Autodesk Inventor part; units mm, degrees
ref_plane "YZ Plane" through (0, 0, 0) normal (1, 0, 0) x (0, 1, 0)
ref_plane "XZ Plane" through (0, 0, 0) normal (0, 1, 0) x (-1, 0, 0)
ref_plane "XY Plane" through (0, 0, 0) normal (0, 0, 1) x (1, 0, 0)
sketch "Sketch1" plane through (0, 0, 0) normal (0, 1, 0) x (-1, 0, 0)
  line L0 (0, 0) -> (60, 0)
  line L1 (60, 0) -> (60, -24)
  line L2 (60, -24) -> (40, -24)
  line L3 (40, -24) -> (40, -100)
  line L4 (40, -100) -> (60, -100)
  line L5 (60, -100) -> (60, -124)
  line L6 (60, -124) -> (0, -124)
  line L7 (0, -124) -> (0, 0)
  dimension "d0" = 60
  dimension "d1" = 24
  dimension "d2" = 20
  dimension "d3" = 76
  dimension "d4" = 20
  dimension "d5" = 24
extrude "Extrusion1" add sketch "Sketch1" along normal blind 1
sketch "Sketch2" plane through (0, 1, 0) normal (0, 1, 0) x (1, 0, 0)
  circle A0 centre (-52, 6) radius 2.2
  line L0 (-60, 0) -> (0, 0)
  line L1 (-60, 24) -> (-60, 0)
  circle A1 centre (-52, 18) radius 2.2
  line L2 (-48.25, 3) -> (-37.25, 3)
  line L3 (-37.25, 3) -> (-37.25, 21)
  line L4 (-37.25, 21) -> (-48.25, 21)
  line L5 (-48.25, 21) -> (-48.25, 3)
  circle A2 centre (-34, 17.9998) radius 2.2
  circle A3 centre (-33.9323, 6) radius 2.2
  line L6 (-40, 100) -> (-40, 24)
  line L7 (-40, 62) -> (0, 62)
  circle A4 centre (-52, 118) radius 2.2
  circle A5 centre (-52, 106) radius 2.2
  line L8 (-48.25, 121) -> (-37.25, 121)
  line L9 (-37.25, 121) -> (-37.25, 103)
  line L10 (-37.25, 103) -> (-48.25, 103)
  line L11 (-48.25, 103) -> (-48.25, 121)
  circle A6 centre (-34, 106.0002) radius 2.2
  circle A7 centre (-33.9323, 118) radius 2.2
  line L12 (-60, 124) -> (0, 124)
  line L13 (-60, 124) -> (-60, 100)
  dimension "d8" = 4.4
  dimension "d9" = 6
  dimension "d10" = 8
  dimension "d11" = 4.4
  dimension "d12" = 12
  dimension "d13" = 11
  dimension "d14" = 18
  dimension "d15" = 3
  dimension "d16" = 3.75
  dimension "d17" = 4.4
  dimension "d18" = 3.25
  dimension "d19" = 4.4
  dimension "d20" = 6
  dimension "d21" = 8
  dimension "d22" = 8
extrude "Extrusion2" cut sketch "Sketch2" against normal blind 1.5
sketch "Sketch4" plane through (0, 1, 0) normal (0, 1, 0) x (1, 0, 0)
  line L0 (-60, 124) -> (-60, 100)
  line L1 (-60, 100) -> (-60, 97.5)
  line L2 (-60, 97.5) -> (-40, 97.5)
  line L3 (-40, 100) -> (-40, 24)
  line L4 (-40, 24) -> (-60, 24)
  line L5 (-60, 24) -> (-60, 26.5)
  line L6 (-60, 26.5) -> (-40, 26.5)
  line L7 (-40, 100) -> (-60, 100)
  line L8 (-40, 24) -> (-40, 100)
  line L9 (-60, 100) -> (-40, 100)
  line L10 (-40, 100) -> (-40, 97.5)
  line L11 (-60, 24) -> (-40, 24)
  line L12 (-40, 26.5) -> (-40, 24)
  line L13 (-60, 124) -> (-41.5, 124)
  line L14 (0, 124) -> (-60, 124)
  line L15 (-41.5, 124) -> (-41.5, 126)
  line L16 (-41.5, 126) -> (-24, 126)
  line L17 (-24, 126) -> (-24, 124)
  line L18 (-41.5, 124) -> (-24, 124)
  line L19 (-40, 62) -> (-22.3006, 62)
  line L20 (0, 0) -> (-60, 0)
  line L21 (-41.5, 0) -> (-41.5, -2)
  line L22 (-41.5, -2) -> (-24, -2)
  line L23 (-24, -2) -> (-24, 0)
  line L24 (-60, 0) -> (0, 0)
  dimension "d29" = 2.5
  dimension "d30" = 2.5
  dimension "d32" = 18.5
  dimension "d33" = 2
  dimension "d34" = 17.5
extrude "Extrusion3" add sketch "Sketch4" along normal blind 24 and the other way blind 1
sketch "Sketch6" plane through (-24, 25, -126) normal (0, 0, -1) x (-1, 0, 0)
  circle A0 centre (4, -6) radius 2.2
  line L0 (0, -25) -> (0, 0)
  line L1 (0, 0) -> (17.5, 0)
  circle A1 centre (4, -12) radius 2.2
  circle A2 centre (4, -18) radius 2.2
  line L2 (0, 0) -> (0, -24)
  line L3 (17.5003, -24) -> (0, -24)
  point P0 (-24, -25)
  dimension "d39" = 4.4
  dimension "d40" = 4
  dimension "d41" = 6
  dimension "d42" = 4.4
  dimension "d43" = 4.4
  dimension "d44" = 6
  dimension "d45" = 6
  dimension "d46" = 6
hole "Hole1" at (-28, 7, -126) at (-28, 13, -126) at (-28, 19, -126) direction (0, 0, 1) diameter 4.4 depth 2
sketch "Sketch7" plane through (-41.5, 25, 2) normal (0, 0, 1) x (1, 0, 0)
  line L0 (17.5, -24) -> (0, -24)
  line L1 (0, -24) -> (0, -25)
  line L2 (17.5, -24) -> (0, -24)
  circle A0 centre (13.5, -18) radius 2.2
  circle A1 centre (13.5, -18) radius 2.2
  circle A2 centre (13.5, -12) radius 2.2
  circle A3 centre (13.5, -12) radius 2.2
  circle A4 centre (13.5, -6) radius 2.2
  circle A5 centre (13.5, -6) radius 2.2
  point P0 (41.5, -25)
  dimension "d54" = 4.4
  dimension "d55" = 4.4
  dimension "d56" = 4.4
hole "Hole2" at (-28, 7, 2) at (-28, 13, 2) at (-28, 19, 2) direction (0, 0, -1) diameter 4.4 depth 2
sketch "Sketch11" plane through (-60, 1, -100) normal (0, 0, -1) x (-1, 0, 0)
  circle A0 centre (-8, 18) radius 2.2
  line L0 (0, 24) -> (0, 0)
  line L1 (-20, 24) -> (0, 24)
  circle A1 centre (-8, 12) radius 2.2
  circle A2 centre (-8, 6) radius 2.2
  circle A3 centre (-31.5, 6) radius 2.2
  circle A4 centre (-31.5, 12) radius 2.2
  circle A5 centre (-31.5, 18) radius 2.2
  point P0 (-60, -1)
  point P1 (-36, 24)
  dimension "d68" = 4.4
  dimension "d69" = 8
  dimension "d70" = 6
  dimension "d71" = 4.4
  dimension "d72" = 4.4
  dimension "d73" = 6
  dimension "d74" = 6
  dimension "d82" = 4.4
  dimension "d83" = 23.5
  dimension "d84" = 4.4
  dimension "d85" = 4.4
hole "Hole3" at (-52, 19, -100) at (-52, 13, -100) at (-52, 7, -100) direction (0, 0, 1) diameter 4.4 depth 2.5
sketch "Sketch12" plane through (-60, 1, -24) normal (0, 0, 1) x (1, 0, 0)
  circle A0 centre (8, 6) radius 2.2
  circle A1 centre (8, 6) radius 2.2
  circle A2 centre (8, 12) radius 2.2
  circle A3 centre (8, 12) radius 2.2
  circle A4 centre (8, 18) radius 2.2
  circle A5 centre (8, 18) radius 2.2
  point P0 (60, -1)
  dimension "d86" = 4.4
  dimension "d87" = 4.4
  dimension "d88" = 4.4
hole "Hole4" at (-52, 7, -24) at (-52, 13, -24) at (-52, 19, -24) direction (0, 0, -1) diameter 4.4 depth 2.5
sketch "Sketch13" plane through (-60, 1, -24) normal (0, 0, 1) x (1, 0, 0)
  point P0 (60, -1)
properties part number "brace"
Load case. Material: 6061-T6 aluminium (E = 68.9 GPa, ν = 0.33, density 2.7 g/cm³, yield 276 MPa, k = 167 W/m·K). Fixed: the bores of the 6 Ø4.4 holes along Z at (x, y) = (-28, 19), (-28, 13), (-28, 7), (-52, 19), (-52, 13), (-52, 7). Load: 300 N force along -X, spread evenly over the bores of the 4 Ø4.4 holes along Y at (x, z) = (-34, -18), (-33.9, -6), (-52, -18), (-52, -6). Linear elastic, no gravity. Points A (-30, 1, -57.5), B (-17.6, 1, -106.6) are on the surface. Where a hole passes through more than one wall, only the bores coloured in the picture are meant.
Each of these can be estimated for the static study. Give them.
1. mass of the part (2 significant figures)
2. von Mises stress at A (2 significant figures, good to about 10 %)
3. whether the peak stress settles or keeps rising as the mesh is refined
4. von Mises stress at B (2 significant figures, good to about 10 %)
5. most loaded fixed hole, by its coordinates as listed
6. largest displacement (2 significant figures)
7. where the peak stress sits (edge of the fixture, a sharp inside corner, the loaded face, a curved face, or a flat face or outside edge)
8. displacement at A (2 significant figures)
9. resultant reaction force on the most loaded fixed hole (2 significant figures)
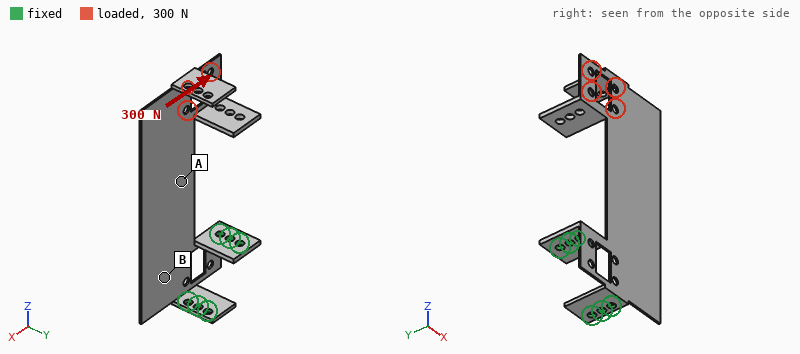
25 g
29 MPa
keeps rising
74 MPa
(-52, 7)
1.1 mm
a sharp inside corner
0.43 mm
1.5 kN
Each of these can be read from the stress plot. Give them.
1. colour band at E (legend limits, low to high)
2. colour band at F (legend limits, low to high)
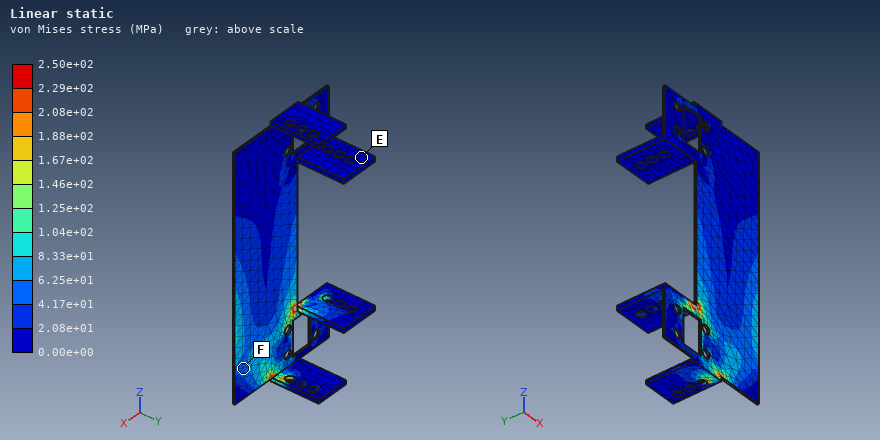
0.00e+00 to 2.08e+01 MPa
4.17e+01 to 6.25e+01 MPa
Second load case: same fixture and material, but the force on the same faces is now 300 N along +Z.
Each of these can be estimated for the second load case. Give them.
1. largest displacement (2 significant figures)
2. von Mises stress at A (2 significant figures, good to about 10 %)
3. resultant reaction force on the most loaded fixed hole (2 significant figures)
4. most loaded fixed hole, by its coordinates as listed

0.24 mm
21 MPa
200 N
(-28, 7)
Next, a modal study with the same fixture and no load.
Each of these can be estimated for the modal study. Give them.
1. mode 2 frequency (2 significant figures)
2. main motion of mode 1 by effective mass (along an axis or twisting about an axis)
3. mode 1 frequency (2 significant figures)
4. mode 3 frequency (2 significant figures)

140 Hz
along Y
44 Hz
260 Hz
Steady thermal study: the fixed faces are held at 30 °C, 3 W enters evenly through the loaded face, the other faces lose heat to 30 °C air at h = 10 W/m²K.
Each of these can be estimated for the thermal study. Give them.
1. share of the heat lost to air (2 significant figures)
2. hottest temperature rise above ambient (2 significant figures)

66 %
34 K
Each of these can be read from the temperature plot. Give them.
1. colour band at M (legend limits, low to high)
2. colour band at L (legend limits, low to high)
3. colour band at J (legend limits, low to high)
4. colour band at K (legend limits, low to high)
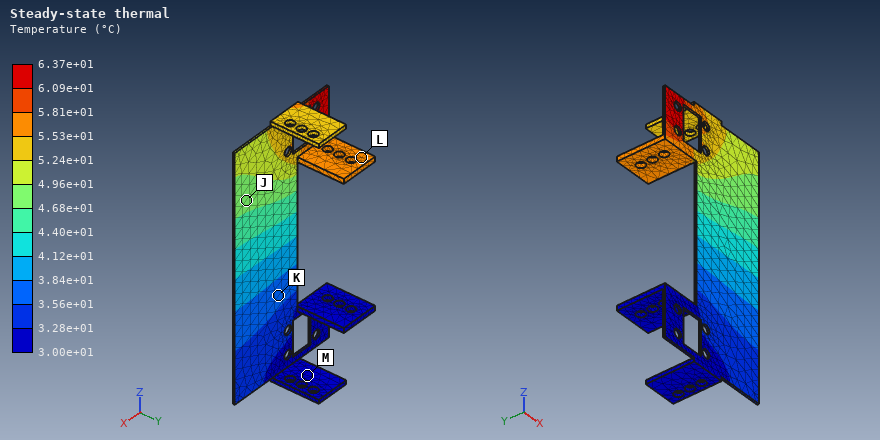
3.00e+01 to 3.28e+01 °C
5.53e+01 to 5.81e+01 °C
4.68e+01 to 4.96e+01 °C
3.56e+01 to 3.84e+01 °C
